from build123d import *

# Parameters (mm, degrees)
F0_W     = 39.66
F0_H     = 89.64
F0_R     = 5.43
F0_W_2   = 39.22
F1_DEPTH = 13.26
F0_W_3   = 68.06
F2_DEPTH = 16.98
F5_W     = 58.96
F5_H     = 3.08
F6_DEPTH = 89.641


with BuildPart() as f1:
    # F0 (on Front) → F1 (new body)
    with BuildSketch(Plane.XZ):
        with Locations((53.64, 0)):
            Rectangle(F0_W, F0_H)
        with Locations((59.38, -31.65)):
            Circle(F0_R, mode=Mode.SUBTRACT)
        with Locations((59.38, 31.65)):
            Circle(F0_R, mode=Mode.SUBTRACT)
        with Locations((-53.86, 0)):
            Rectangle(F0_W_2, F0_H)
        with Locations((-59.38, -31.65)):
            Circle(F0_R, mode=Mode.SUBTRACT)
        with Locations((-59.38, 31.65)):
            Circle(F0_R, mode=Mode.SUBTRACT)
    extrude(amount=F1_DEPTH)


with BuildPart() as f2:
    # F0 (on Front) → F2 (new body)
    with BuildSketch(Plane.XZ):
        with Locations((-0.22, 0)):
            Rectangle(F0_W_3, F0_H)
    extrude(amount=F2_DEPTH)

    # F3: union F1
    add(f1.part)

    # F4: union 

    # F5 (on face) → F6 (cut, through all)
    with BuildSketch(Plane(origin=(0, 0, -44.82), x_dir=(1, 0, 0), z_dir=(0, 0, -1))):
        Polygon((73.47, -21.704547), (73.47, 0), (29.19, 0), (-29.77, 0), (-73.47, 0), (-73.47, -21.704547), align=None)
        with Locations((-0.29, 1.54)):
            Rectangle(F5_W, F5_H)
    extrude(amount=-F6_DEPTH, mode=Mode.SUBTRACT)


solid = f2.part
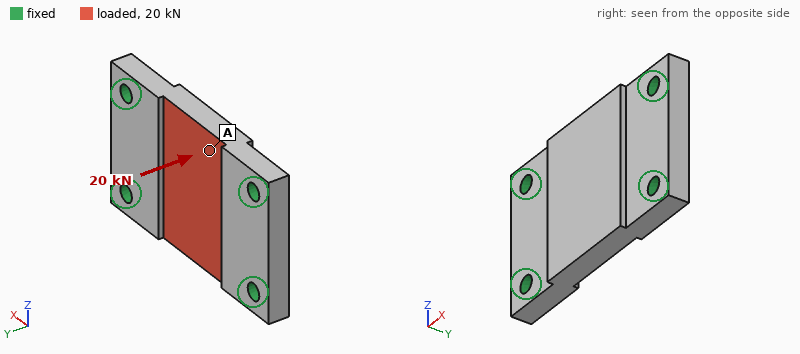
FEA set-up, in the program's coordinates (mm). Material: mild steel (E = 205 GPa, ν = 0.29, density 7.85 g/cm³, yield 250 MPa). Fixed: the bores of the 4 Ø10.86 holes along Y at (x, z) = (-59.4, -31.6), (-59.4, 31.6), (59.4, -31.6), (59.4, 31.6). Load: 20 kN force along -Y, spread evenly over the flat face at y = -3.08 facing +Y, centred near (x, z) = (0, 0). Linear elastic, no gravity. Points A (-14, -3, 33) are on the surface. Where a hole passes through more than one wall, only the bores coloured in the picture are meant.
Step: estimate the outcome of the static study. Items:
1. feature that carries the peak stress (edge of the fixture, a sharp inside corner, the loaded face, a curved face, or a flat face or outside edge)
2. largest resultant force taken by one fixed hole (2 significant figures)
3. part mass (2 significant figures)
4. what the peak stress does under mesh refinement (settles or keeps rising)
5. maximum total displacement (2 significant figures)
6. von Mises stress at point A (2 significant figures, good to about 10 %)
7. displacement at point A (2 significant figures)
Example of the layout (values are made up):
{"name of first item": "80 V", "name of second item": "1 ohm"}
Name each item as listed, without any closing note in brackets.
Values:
{"feature that carries the peak stress": "edge of the fixture", "largest resultant force taken by one fixed hole": "7.2 kN", "part mass": "1.4 kg", "what the peak stress does under mesh refinement": "keeps rising", "maximum total displacement": "40 µm", "von Mises stress at point A": "36 MPa", "displacement at point A": "35 µm"}
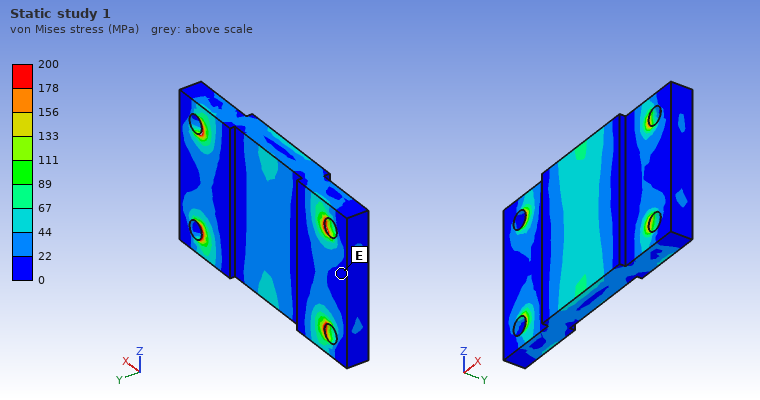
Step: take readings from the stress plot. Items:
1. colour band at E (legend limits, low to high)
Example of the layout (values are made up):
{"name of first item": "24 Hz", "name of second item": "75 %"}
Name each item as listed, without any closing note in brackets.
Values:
{"colour band at E": "0 to 22 MPa"}
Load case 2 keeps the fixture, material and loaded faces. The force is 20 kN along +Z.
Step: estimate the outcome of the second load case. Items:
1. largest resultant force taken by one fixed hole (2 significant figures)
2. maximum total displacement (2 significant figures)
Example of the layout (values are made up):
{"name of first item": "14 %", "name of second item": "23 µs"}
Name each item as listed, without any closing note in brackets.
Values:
{"largest resultant force taken by one fixed hole": "5.9 kN", "maximum total displacement": "11 µm"}
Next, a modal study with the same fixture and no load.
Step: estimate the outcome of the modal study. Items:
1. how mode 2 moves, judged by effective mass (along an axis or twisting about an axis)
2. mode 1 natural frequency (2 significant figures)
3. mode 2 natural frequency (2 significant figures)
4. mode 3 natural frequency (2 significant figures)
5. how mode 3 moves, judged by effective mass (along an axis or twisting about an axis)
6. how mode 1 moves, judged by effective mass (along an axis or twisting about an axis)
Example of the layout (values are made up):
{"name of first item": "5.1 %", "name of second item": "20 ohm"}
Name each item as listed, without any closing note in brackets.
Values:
{"how mode 2 moves, judged by effective mass": "twisting about X", "mode 1 natural frequency": "4700 Hz", "mode 2 natural frequency": "6400 Hz", "mode 3 natural frequency": "11 kHz", "how mode 3 moves, judged by effective mass": "twisting about Z", "how mode 1 moves, judged by effective mass": "along Y"}
